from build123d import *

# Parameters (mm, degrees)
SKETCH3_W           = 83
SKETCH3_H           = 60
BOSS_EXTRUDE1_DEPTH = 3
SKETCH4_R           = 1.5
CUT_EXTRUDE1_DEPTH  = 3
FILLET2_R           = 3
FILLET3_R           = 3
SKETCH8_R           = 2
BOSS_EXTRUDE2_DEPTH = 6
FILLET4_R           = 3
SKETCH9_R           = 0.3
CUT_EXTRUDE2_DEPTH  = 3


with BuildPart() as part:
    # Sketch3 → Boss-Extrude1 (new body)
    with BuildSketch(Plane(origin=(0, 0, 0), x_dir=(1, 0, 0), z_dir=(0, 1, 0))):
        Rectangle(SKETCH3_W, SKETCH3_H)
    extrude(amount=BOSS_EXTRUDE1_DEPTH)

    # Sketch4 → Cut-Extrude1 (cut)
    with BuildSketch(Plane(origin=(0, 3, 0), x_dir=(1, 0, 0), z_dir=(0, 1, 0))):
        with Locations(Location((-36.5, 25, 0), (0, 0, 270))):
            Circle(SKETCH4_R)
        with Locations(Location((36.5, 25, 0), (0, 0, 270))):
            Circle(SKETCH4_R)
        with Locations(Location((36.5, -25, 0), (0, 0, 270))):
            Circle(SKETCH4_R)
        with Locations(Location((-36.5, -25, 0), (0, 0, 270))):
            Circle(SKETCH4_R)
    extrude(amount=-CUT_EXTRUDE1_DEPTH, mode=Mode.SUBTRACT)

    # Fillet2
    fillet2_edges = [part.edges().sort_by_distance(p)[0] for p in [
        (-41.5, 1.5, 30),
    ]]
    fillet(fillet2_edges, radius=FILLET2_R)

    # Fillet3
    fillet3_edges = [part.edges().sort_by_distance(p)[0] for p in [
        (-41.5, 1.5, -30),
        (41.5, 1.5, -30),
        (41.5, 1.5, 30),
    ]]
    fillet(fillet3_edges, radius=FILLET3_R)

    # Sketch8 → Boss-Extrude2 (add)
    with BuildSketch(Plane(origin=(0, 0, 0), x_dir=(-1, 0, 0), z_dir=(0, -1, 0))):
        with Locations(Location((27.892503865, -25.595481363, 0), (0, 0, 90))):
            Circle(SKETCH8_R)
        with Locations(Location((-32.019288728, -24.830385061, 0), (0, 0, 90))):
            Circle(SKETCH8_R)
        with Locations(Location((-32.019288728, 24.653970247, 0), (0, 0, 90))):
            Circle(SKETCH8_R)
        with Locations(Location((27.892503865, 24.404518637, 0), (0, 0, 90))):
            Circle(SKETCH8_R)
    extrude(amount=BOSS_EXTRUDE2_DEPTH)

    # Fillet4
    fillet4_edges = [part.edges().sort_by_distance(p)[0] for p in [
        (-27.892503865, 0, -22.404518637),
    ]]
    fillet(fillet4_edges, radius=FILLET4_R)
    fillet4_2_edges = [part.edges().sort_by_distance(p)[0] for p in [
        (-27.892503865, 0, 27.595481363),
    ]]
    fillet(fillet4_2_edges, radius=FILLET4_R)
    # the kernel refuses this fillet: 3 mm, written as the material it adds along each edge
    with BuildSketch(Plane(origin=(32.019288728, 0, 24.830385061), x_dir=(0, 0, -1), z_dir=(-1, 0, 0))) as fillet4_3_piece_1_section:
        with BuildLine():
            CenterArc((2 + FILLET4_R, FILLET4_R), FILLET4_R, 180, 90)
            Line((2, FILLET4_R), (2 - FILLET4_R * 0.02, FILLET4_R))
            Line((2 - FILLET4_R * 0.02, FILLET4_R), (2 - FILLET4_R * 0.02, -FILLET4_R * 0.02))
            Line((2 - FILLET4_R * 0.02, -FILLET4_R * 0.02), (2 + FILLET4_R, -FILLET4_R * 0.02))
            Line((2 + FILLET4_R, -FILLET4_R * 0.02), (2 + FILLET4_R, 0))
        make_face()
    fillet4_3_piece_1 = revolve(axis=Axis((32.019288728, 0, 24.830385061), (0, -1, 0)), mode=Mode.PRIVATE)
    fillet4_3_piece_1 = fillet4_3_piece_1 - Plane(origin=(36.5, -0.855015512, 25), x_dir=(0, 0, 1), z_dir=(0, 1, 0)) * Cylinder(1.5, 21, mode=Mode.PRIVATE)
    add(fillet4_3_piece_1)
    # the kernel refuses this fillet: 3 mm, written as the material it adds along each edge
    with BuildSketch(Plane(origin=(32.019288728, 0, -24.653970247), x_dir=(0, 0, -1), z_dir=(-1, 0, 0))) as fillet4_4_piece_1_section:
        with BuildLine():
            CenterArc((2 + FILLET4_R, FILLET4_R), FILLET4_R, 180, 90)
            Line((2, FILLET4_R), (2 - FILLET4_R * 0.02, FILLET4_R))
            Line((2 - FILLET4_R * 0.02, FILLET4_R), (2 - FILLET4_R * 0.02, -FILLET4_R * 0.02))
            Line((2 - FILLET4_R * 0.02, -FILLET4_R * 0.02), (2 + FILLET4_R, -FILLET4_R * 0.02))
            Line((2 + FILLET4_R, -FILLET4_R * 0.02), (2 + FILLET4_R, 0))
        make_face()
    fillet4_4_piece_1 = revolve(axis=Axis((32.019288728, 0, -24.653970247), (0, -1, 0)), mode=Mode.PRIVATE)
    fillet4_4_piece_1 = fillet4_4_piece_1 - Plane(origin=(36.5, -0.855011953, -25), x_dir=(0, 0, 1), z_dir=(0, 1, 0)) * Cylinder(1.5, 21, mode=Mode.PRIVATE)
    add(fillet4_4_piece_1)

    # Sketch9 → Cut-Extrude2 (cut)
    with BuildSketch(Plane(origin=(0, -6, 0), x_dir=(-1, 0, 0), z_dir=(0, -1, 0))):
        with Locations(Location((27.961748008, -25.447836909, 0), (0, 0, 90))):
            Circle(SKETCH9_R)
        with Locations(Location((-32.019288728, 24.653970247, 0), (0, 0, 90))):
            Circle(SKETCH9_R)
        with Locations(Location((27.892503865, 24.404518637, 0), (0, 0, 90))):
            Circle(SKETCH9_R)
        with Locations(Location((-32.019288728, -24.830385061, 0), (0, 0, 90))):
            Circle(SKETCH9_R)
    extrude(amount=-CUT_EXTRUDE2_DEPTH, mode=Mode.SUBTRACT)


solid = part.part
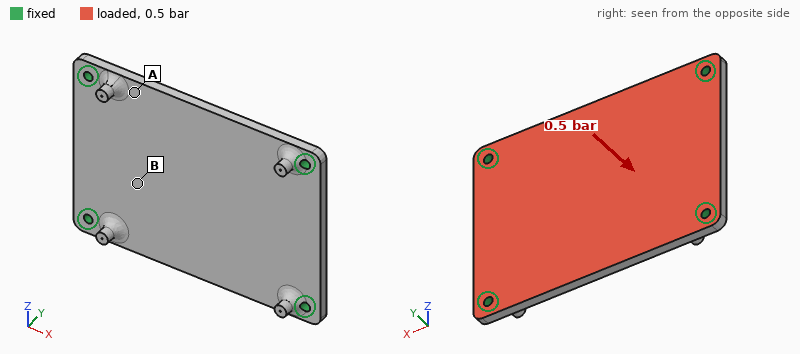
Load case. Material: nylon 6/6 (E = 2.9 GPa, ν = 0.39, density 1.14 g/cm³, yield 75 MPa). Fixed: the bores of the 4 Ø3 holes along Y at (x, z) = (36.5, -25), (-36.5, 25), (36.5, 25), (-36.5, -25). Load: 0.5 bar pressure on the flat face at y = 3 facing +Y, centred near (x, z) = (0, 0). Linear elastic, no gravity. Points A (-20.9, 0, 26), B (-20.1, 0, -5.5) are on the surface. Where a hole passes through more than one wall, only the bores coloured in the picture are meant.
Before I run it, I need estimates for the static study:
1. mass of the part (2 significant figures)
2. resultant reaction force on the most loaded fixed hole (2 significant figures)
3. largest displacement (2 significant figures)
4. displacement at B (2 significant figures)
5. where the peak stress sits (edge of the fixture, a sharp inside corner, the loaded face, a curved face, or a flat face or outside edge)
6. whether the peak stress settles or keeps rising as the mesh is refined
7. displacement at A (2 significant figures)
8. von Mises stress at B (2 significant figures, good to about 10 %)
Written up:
17 g
66 N
0.79 mm
0.54 mm
edge of the fixture
keeps rising
0.34 mm
4.5 MPa
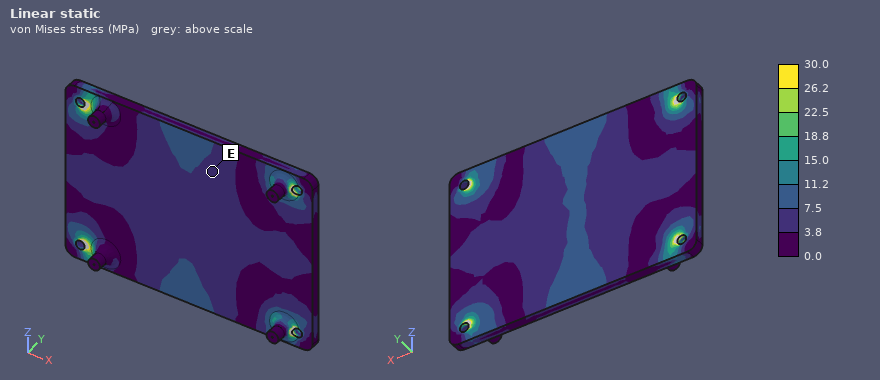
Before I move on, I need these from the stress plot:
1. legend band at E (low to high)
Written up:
3.8 to 7.5 MPa
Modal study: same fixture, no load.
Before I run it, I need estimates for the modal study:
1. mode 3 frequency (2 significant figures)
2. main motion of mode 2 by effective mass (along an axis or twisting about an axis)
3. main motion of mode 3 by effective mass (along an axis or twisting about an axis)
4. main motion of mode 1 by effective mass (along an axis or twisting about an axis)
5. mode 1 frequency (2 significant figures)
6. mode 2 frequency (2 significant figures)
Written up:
1800 Hz
twisting about X
twisting about Z
along Y
800 Hz
1200 Hz
